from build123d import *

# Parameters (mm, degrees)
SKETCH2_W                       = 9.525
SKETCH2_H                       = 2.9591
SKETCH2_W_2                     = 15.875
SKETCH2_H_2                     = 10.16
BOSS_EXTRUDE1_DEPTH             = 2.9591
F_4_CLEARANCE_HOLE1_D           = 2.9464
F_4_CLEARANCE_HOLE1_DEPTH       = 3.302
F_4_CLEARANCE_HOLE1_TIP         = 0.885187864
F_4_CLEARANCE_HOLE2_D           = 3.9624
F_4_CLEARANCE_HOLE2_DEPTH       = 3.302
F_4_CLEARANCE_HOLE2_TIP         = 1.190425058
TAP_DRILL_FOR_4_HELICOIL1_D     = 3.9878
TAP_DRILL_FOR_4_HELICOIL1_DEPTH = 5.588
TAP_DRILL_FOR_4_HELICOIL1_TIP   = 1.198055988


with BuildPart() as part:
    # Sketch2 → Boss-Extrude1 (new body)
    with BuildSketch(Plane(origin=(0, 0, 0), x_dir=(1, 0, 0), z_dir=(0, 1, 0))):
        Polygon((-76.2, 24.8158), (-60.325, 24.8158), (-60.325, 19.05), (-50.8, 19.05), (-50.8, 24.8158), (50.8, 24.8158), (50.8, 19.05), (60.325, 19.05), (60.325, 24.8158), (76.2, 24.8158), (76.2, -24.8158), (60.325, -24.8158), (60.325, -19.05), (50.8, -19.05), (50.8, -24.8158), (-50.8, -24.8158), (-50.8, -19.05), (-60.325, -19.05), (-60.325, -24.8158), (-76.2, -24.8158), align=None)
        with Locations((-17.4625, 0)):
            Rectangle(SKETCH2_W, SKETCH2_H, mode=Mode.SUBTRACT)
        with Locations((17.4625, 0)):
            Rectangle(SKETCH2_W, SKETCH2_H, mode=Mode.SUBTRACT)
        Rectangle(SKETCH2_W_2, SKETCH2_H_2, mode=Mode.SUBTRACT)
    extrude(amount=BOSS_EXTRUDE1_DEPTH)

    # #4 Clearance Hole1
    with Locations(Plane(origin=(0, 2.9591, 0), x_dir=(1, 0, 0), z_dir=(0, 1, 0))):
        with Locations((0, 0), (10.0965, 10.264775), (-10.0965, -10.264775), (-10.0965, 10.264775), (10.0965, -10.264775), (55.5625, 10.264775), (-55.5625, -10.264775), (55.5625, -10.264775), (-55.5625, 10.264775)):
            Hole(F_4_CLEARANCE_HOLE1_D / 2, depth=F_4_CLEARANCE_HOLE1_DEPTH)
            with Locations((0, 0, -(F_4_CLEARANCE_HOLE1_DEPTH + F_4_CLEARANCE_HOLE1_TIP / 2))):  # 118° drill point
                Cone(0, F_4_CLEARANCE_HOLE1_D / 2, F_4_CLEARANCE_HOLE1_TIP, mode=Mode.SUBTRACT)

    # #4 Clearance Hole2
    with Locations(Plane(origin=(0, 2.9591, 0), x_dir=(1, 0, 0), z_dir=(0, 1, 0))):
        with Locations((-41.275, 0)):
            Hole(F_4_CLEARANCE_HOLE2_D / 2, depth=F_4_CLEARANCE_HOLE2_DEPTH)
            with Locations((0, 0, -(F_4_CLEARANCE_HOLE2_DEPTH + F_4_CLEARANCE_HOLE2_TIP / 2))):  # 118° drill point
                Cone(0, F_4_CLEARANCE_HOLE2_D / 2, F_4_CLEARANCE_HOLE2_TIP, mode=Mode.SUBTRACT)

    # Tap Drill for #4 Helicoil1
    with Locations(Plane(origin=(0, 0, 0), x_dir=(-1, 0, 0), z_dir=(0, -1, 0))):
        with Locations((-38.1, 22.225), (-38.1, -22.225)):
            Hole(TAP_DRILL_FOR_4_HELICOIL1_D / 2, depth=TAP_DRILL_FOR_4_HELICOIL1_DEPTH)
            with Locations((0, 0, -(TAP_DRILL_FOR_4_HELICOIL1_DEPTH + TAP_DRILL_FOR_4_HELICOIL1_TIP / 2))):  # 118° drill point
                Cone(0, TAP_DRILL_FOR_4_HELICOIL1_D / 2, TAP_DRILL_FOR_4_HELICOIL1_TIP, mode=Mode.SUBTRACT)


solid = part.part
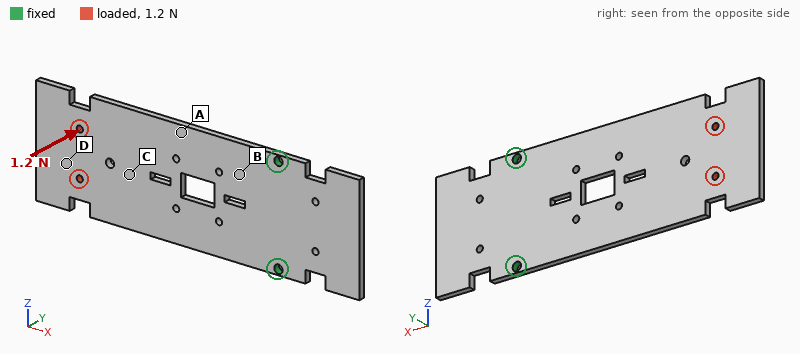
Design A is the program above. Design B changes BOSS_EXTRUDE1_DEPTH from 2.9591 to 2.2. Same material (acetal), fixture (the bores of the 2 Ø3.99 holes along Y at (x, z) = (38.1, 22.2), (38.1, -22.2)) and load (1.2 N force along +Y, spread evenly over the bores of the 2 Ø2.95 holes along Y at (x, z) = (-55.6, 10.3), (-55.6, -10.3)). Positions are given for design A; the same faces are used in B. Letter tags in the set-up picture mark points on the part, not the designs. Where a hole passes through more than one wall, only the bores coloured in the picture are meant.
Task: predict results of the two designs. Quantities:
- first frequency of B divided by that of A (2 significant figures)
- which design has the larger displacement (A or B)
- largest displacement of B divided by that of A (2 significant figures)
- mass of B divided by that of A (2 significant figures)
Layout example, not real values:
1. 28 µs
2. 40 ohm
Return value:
1. 0.75
2. B
3. 2.4
4. 0.74
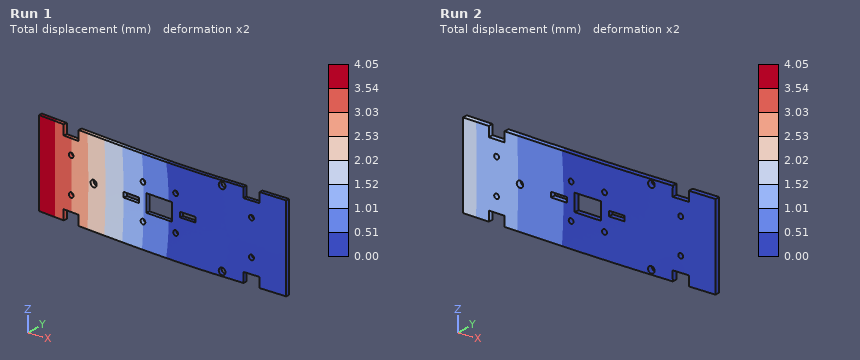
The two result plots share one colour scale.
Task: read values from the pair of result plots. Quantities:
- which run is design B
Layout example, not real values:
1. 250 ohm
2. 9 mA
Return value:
1. Run 1
